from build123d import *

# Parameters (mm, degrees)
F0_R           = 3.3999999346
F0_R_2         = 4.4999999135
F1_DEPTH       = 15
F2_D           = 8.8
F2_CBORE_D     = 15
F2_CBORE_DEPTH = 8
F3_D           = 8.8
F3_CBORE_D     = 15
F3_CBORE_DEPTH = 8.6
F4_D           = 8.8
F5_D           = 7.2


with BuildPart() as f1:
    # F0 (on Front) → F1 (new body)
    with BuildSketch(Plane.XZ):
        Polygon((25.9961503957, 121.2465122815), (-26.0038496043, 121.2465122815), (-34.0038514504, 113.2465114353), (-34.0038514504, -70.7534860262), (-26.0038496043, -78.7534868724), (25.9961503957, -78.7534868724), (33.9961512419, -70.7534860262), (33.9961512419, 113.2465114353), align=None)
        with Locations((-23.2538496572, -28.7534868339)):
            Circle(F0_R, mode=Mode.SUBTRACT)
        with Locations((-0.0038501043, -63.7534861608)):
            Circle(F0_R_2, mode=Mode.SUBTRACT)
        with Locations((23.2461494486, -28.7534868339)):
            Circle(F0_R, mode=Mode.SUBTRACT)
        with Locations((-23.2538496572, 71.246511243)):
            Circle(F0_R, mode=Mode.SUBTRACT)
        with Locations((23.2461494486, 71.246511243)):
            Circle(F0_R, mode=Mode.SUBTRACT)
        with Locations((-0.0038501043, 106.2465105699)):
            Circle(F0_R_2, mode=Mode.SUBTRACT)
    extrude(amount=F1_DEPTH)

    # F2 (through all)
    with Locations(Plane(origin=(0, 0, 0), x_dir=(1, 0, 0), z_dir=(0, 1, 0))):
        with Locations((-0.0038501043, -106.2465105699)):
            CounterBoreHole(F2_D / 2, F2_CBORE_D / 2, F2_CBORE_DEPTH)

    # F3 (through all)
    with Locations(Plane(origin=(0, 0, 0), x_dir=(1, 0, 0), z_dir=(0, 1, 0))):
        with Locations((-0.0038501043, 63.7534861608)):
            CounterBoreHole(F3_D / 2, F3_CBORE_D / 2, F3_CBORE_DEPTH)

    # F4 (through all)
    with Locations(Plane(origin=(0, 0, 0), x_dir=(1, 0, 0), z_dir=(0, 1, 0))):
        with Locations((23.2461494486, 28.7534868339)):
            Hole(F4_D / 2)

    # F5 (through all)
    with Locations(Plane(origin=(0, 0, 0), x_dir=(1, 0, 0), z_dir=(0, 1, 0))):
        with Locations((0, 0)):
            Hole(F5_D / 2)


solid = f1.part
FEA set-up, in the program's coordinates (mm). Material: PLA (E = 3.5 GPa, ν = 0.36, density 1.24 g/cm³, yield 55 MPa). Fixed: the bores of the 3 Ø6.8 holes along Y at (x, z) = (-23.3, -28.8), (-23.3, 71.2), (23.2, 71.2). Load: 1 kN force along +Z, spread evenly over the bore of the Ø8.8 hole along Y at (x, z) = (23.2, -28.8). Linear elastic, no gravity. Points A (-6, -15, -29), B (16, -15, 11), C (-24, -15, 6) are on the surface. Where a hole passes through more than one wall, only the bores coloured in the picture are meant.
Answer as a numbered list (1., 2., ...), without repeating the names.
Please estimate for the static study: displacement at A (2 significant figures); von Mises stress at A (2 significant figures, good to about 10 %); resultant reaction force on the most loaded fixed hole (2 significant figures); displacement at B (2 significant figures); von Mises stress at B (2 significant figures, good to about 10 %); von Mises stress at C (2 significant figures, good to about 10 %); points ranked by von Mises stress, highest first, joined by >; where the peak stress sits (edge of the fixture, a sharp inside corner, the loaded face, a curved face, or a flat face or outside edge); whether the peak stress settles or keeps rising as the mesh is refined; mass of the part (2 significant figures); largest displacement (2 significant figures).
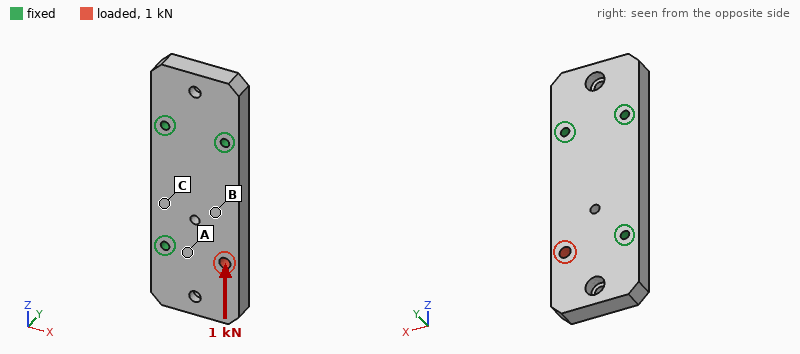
1. 15 µm
2. 0.68 MPa
3. 420 N
4. 22 µm
5. 1.5 MPa
6. 0.42 MPa
7. B > A > C
8. edge of the fixture
9. keeps rising
10. 240 g
11. 73 µm
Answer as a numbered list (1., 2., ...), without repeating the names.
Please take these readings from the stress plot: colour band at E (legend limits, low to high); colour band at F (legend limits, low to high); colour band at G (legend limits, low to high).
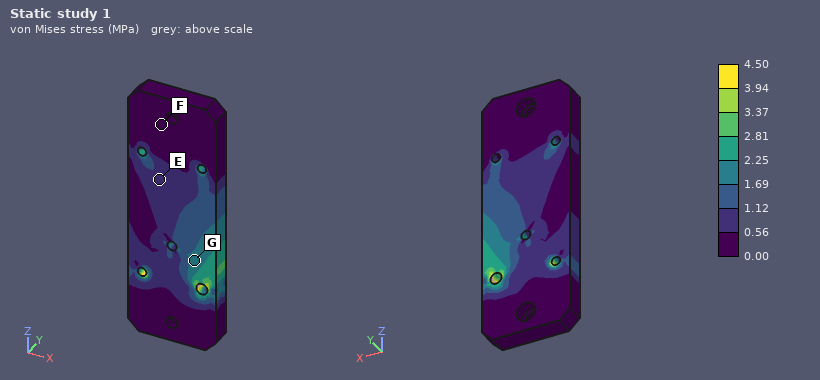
1. 0.56 to 1.12 MPa
2. 0.00 to 0.56 MPa
3. 1.69 to 2.25 MPa
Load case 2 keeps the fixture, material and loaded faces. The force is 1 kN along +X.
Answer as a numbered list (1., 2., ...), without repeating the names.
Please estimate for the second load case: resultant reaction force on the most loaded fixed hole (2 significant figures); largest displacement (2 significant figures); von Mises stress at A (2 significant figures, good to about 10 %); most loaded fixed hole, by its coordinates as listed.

1. 940 N
2. 42 µm
3. 2.4 MPa
4. (-23.3, -28.8)
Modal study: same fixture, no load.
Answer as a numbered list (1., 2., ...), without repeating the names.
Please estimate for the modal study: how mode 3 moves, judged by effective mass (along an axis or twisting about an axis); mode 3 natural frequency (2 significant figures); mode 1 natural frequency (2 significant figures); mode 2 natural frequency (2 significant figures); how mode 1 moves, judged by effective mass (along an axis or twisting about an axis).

1. along Y
2. 1500 Hz
3. 870 Hz
4. 1300 Hz
5. along Y
